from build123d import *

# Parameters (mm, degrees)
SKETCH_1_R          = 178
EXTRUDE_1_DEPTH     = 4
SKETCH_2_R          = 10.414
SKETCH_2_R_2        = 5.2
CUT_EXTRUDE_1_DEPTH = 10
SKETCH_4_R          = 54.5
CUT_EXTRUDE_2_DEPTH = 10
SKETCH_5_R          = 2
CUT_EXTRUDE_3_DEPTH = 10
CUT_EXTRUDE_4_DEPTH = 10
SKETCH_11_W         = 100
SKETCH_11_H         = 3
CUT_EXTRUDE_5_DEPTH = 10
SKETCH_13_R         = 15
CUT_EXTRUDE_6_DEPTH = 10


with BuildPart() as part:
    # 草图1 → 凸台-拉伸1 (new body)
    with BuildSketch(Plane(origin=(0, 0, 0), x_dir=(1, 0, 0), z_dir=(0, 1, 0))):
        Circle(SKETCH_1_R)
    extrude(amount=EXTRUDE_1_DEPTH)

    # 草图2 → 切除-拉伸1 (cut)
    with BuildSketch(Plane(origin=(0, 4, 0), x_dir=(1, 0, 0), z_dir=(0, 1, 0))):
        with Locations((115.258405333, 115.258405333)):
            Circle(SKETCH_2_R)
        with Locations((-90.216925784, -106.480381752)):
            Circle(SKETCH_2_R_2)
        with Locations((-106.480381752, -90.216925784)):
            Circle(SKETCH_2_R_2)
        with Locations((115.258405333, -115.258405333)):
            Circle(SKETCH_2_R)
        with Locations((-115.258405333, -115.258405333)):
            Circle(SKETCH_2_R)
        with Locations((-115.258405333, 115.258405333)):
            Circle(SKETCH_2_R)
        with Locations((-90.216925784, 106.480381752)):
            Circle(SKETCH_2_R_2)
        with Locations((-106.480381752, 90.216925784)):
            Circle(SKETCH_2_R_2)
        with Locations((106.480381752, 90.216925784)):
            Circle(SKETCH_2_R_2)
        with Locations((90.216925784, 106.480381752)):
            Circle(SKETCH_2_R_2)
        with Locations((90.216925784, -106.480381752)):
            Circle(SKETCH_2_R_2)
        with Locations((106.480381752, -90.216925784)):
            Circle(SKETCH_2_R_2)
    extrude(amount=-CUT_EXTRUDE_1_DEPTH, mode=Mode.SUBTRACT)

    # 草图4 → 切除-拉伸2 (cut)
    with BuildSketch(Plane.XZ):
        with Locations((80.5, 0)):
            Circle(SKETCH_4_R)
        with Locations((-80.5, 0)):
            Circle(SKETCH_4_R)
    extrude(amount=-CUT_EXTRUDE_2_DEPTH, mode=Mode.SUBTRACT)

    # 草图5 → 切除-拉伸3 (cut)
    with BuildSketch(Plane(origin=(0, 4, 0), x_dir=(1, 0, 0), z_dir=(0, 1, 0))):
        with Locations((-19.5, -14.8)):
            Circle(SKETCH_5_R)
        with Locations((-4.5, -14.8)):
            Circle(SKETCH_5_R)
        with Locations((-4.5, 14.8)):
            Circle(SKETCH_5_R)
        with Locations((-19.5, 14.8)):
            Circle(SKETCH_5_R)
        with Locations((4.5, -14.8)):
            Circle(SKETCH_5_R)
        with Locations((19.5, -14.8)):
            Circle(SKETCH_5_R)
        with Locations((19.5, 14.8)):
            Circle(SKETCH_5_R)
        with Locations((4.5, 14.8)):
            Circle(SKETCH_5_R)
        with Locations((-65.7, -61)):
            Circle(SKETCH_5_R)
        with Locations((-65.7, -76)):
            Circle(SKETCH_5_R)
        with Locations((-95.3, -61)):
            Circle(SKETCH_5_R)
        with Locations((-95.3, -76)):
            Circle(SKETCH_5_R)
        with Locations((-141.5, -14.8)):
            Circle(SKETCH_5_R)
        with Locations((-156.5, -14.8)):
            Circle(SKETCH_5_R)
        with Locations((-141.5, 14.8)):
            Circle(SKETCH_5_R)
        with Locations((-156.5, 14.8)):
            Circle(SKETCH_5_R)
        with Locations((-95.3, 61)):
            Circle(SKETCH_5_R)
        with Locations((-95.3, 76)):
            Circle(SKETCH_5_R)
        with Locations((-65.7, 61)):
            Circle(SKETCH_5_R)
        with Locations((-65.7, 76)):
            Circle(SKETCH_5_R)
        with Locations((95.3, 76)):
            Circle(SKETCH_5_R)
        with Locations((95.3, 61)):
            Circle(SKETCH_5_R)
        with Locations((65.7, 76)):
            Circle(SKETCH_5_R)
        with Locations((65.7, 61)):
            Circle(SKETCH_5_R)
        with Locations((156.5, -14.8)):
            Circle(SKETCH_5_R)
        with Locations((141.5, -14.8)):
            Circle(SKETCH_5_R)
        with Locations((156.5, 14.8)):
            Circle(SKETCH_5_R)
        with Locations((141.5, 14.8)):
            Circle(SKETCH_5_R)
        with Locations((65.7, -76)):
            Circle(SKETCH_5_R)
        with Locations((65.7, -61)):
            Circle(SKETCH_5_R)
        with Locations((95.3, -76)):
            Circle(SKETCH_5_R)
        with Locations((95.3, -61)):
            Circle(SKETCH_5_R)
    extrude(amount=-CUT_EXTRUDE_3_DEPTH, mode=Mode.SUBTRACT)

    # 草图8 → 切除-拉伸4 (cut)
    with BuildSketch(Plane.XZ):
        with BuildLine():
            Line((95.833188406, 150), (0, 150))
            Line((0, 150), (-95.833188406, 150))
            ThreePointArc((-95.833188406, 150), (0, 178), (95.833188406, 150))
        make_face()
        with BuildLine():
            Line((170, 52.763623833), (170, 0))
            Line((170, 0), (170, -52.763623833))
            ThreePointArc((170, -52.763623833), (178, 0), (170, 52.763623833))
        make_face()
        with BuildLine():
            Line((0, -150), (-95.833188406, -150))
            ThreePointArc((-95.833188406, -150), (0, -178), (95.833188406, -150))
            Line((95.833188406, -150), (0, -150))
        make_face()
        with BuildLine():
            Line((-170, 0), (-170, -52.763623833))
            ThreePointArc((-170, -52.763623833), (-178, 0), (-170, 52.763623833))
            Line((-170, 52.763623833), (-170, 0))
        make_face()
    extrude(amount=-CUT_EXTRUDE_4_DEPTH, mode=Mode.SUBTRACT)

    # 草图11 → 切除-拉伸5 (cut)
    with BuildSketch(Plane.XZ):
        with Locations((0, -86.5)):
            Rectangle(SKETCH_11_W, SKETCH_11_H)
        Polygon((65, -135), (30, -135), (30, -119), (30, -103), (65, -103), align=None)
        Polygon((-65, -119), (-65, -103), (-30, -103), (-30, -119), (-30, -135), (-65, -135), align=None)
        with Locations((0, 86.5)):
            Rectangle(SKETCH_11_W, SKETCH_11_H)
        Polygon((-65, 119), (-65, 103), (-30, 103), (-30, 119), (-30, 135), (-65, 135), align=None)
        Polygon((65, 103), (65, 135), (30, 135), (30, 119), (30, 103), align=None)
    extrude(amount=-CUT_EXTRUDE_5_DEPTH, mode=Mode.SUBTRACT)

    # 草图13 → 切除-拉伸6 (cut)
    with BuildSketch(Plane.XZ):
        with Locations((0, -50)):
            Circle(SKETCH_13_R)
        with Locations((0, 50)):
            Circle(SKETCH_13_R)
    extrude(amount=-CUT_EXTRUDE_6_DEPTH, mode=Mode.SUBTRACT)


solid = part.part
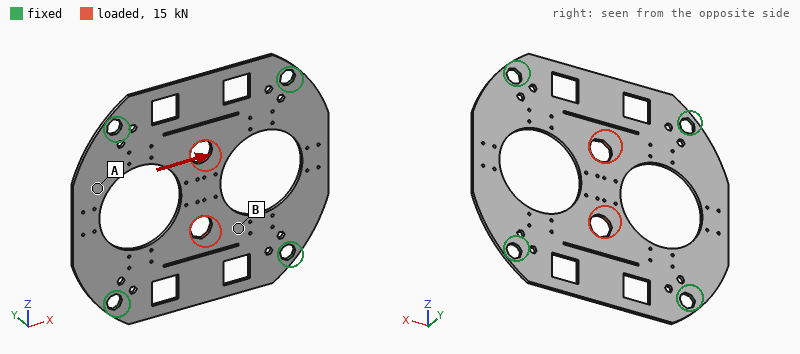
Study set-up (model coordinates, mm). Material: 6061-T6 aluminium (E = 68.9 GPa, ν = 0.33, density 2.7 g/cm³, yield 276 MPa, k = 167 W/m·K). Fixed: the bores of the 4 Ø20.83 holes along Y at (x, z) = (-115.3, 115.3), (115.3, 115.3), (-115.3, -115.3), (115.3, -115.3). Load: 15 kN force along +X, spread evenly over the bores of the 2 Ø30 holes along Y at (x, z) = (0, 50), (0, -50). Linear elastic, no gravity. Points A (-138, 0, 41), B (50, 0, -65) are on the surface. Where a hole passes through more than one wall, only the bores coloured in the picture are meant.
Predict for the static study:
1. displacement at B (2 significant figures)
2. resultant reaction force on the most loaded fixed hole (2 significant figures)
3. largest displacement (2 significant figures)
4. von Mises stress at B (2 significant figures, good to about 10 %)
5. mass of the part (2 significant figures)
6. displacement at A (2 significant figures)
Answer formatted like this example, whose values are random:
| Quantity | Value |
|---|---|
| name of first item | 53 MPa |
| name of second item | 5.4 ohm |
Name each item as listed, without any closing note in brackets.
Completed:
| Quantity | Value |
|---|---|
| displacement at B | 34 µm |
| resultant reaction force on the most loaded fixed hole | 3.9 kN |
| largest displacement | 59 µm |
| von Mises stress at B | 21 MPa |
| mass of the part | 690 g |
| displacement at A | 21 µm |
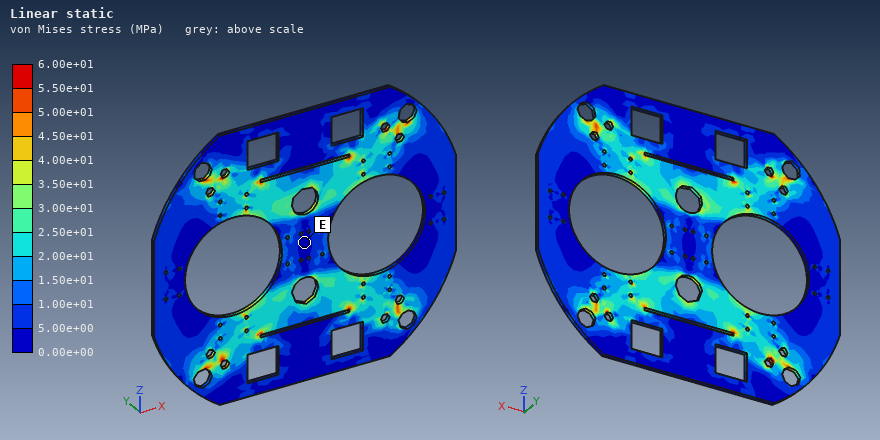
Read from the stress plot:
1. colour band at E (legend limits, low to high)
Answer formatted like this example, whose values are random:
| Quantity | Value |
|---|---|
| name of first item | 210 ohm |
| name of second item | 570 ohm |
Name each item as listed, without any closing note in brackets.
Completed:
| Quantity | Value |
|---|---|
| colour band at E | 0.00e+00 to 5.00e+00 MPa |
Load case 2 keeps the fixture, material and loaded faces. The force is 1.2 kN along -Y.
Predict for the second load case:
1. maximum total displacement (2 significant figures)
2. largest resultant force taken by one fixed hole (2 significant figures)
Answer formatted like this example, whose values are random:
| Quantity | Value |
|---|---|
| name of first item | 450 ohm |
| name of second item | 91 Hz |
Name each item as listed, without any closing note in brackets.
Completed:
| Quantity | Value |
|---|---|
| maximum total displacement | 2.7 mm |
| largest resultant force taken by one fixed hole | 300 N |
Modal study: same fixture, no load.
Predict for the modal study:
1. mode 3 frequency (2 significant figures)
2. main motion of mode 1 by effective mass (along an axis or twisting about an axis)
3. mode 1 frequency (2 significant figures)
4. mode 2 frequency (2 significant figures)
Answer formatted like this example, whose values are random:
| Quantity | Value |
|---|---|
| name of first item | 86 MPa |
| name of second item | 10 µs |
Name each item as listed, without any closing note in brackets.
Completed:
| Quantity | Value |
|---|---|
| mode 3 frequency | 420 Hz |
| main motion of mode 1 by effective mass | along Y |
| mode 1 frequency | 300 Hz |
| mode 2 frequency | 410 Hz |
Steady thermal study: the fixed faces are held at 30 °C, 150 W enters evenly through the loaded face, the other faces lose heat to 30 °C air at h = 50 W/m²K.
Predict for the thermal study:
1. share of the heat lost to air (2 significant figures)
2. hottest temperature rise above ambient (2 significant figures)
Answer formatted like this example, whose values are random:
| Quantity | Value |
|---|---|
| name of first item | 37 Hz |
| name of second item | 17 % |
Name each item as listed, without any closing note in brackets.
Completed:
| Quantity | Value |
|---|---|
| share of the heat lost to air | 73 % |
| hottest temperature rise above ambient | 70 K |
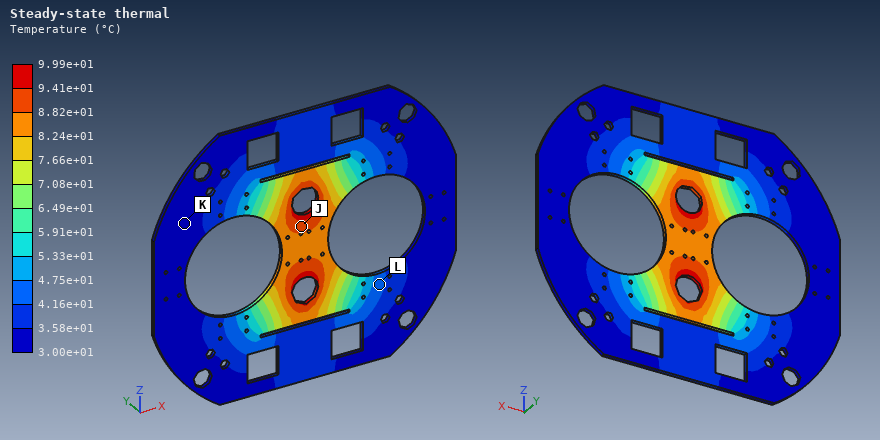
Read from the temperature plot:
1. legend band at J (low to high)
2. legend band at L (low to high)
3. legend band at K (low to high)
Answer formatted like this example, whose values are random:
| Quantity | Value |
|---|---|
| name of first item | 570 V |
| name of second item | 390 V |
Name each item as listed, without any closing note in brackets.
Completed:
| Quantity | Value |
|---|---|
| legend band at J | 8.82e+01 to 9.41e+01 °C |
| legend band at L | 4.16e+01 to 4.75e+01 °C |
| legend band at K | 3.00e+01 to 3.58e+01 °C |
